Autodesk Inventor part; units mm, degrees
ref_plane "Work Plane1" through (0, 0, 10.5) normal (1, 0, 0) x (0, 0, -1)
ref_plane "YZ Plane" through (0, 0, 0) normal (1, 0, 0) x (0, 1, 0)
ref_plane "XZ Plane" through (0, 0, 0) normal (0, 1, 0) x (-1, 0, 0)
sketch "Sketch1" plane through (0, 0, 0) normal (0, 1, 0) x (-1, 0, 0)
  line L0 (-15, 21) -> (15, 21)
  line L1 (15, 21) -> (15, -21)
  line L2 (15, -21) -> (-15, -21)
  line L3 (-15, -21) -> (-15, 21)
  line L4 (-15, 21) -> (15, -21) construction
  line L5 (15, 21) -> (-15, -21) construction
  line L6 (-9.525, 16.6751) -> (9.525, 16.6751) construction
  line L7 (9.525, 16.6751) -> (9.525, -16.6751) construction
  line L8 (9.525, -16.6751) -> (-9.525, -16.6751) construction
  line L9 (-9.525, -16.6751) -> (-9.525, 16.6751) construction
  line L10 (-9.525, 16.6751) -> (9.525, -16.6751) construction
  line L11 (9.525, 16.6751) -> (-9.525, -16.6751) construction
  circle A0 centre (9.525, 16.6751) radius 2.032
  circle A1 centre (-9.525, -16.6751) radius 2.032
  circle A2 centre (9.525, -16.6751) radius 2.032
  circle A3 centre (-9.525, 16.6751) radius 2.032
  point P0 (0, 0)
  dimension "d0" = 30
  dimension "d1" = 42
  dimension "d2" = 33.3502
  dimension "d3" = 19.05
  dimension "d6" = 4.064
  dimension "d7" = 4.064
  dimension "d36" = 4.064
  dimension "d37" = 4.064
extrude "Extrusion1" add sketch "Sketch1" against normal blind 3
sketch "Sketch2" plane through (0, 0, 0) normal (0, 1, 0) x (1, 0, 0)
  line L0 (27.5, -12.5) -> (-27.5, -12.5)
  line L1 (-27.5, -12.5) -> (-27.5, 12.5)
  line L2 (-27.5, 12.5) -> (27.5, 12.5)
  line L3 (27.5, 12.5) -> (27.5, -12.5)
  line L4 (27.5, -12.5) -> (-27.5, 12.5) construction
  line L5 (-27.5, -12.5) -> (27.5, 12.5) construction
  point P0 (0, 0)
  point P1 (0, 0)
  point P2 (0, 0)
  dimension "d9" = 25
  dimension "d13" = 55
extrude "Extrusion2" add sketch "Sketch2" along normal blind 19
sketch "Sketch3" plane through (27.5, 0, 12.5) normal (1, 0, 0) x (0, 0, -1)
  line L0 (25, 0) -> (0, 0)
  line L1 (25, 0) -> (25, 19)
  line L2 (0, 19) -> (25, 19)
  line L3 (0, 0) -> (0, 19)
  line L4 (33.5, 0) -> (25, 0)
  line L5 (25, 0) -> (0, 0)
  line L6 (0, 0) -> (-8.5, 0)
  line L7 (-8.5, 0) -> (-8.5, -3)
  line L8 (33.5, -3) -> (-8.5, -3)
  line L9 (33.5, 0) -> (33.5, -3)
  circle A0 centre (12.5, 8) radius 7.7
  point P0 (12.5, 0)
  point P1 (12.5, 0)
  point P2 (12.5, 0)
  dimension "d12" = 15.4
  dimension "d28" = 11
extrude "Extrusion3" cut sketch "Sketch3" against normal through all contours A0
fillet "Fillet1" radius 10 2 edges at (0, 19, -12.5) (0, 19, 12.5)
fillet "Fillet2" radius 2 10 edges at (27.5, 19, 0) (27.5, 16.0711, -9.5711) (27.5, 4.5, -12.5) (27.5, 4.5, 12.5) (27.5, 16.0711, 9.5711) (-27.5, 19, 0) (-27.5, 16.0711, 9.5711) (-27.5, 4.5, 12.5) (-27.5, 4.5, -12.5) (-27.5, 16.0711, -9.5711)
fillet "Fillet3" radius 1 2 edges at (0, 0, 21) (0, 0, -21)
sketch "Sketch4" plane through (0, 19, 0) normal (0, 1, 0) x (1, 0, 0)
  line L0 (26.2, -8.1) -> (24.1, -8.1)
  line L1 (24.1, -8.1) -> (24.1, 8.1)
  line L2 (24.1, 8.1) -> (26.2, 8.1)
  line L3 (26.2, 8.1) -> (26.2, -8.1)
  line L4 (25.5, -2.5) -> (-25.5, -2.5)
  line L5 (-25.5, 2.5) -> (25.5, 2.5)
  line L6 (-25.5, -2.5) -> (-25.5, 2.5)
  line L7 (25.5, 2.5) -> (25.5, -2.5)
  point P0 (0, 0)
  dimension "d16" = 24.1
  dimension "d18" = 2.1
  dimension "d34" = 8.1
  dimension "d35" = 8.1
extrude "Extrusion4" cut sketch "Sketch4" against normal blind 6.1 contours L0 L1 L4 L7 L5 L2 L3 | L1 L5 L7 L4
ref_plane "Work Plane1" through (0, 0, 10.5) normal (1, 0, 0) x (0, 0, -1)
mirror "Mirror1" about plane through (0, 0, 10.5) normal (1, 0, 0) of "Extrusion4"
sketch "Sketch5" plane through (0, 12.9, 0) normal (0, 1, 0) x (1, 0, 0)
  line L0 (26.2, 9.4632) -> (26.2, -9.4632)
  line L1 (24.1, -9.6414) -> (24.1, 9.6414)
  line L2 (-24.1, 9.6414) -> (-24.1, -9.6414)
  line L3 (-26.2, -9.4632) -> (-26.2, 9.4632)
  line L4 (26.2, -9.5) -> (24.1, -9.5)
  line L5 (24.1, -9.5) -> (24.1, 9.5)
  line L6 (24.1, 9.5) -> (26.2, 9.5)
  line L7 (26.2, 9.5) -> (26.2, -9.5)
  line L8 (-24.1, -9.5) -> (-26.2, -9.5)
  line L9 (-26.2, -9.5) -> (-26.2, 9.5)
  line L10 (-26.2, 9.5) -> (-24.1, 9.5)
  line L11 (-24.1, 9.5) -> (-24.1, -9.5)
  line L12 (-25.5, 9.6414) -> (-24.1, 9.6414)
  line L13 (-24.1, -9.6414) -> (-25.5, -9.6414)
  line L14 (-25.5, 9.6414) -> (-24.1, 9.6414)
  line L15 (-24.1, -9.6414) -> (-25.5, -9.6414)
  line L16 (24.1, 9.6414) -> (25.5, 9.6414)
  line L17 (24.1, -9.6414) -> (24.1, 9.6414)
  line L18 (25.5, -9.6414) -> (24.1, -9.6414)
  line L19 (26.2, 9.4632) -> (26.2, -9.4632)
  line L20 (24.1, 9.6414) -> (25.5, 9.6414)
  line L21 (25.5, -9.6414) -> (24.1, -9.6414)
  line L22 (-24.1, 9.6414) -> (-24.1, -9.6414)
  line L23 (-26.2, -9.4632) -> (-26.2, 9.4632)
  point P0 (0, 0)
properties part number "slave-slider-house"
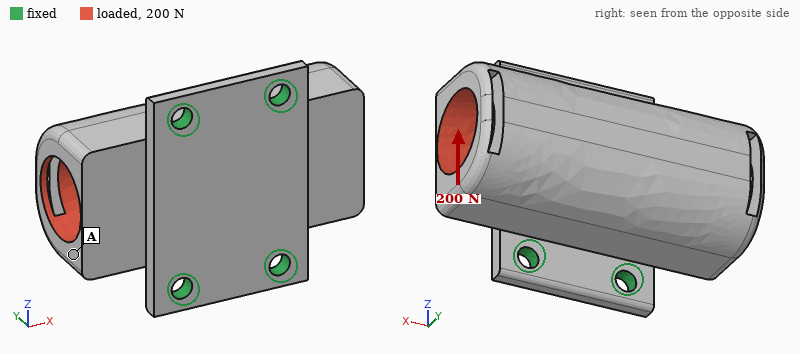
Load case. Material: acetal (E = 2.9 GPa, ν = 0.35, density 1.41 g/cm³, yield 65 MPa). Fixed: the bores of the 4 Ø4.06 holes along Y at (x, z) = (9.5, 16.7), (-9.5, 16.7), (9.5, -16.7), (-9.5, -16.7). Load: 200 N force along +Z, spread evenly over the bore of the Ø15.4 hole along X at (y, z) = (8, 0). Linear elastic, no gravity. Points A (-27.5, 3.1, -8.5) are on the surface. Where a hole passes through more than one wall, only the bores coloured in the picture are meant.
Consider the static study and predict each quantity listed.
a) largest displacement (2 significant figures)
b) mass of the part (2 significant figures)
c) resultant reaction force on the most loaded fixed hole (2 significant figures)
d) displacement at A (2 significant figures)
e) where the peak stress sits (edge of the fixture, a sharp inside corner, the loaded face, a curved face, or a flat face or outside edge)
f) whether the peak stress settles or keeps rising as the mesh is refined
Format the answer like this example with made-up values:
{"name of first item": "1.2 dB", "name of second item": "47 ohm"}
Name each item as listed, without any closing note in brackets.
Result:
{"largest displacement": "30 µm", "mass of the part": "24 g", "resultant reaction force on the most loaded fixed hole": "60 N", "displacement at A": "15 µm", "where the peak stress sits": "edge of the fixture", "whether the peak stress settles or keeps rising as the mesh is refined": "keeps rising"}
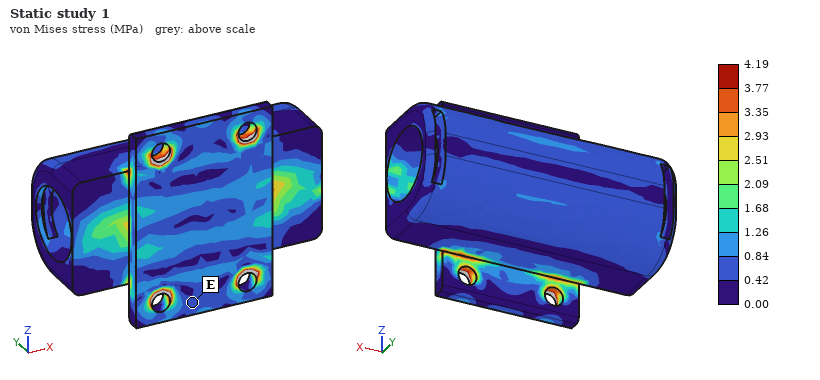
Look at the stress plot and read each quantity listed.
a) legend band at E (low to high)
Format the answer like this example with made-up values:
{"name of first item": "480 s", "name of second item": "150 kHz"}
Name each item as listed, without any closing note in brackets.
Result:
{"legend band at E": "0.42 to 0.84 MPa"}
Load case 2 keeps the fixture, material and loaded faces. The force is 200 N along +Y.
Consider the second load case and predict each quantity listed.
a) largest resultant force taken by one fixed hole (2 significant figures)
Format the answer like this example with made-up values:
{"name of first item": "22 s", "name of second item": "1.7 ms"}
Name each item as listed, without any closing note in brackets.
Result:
{"largest resultant force taken by one fixed hole": "54 N"}
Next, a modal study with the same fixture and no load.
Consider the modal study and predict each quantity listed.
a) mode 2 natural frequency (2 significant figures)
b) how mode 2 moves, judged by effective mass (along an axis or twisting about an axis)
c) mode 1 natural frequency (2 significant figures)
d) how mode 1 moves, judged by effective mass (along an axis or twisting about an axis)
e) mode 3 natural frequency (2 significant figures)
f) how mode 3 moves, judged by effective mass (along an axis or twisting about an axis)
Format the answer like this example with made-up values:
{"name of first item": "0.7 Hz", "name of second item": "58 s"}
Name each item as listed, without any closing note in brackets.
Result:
{"mode 2 natural frequency": "3300 Hz", "how mode 2 moves, judged by effective mass": "along Z", "mode 1 natural frequency": "2000 Hz", "how mode 1 moves, judged by effective mass": "along X", "mode 3 natural frequency": "3700 Hz", "how mode 3 moves, judged by effective mass": "along Y"}
